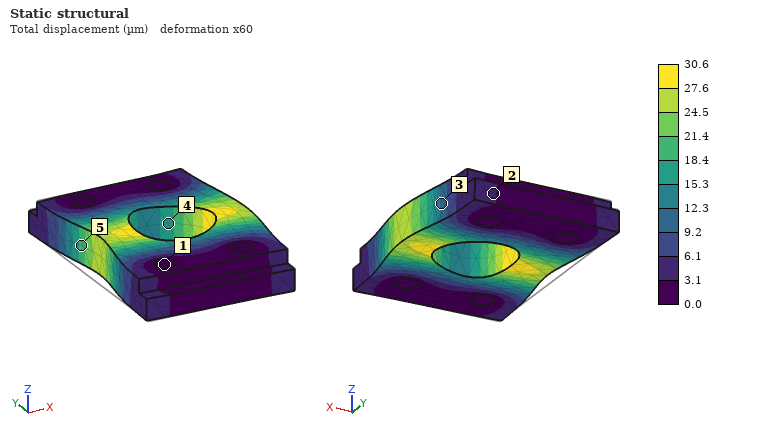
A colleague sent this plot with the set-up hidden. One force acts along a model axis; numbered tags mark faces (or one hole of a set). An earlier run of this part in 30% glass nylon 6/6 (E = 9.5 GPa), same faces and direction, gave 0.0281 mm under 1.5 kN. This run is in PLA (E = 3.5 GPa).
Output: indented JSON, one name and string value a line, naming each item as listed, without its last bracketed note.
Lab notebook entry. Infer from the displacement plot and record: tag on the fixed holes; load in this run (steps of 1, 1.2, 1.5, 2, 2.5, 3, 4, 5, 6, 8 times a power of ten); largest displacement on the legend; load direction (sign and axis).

{
  "tag on the fixed holes": "1",
  "load in this run": "600 N",
  "largest displacement on the legend": "30.6 µm",
  "load direction": "+X"
}
